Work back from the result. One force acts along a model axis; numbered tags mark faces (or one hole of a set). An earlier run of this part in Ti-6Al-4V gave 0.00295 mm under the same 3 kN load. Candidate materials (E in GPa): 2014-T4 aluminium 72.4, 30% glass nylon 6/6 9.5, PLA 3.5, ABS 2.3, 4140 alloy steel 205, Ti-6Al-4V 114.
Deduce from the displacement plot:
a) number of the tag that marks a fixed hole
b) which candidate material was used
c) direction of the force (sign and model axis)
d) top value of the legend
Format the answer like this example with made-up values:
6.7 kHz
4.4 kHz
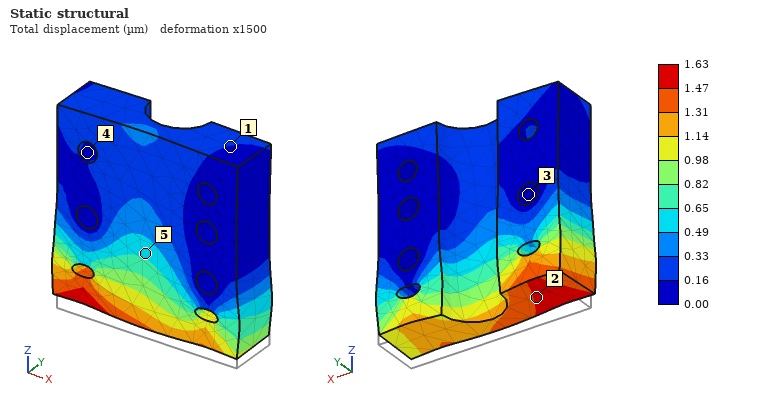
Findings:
3
4140 alloy steel
+Z
1.63 µm
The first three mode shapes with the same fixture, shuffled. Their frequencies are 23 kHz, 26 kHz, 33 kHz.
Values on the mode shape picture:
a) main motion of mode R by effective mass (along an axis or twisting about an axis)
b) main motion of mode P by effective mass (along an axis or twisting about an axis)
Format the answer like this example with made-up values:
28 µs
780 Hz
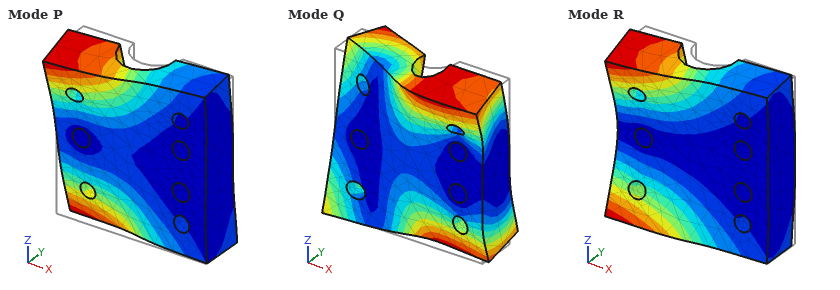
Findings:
along Y
twisting about X
